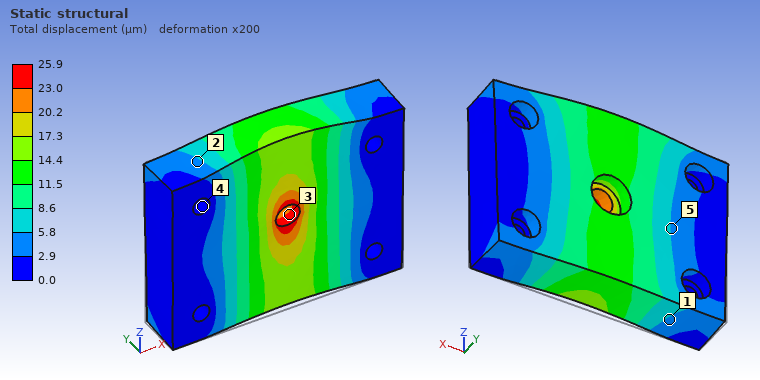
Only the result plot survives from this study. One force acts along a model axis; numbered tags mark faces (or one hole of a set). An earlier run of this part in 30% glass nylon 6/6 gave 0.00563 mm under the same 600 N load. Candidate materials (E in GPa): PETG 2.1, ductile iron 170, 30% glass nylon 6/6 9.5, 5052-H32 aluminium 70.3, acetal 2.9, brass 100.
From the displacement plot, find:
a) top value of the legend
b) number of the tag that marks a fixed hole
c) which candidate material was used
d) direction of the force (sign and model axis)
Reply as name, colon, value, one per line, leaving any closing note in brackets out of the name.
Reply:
top value of the legend: 25.9 µm
number of the tag that marks a fixed hole: 4
which candidate material was used: PETG
direction of the force: +Z
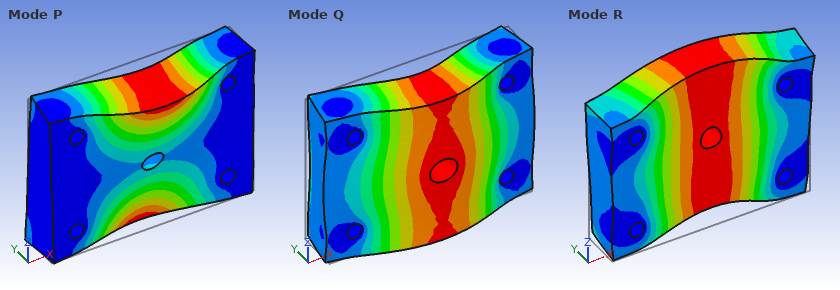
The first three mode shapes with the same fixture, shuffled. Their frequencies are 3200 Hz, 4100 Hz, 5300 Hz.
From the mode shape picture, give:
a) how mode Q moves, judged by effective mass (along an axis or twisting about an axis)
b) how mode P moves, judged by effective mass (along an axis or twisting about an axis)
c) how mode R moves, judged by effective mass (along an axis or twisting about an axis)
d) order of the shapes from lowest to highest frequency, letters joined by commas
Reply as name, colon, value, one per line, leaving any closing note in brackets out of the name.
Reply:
how mode Q moves, judged by effective mass: along Y
how mode P moves, judged by effective mass: twisting about X
how mode R moves, judged by effective mass: along Z
order of the shapes from lowest to highest frequency, letters joined by commas: Q, P, R
